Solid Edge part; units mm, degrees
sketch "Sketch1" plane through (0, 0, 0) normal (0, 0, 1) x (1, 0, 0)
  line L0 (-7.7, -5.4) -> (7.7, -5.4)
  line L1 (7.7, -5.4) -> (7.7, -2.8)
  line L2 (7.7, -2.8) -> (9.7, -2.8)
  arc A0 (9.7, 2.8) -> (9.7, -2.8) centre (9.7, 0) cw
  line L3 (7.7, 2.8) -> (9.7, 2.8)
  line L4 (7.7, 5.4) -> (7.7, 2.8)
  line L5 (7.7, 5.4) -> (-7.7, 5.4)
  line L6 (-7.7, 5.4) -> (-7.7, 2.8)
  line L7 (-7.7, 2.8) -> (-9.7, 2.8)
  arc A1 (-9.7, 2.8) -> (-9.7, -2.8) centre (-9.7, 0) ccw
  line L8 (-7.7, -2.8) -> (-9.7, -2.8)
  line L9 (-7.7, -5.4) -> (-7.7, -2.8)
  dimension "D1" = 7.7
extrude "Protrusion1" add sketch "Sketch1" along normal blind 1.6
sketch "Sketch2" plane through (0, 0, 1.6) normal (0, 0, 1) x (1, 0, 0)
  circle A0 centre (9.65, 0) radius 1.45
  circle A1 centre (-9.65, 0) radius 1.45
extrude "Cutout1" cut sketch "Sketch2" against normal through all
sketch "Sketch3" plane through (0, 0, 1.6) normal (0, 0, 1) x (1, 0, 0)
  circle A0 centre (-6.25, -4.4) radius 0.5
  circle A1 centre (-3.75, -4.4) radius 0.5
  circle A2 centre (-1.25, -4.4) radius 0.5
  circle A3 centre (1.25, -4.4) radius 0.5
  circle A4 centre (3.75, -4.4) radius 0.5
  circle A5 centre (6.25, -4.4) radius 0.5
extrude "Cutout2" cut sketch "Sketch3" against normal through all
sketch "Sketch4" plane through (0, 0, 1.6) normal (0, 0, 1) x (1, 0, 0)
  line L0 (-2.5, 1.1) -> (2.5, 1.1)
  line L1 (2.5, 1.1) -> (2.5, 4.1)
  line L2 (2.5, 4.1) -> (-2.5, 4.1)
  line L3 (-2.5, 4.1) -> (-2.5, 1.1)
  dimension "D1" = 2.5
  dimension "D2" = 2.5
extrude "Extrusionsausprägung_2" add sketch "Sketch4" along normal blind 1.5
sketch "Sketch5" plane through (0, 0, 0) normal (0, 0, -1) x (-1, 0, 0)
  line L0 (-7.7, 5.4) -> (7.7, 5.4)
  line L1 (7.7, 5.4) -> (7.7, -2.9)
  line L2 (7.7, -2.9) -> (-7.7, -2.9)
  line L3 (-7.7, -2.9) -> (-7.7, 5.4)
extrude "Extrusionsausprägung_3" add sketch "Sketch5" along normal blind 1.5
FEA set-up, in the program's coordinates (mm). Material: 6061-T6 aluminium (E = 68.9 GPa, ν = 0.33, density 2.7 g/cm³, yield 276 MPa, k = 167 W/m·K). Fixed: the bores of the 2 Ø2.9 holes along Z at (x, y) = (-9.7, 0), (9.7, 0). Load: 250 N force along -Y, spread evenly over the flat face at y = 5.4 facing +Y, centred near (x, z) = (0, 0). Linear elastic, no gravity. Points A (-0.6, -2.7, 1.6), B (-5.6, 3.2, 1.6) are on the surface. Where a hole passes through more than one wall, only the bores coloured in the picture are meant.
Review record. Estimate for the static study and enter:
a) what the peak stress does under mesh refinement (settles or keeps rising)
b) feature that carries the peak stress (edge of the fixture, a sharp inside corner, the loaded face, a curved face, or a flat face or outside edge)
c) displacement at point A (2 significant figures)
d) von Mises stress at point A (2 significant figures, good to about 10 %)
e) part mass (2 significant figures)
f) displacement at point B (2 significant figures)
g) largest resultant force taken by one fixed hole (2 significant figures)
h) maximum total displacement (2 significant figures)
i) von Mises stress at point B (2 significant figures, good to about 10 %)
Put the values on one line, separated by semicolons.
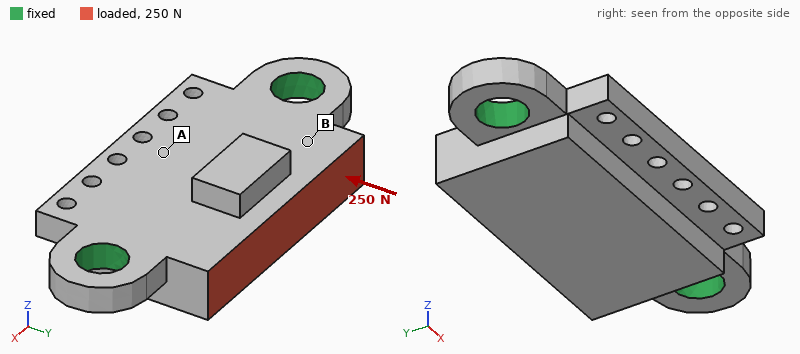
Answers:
keeps rising; edge of the fixture; 2.0 µm; 5.8 MPa; 1.4 g; 2.1 µm; 130 N; 5.0 µm; 10 MPa
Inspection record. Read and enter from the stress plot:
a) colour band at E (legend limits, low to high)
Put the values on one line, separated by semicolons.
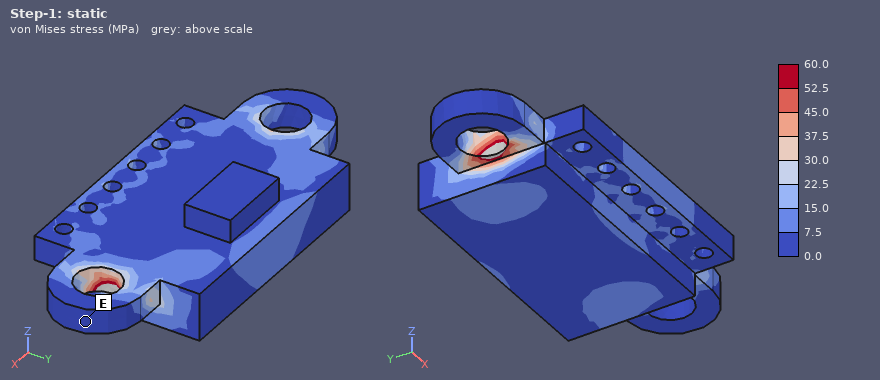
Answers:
0.0 to 7.5 MPa
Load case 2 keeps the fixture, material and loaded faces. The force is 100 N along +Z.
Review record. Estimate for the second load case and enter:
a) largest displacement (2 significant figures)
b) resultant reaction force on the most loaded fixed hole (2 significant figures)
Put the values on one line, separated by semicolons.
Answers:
15 µm; 66 N
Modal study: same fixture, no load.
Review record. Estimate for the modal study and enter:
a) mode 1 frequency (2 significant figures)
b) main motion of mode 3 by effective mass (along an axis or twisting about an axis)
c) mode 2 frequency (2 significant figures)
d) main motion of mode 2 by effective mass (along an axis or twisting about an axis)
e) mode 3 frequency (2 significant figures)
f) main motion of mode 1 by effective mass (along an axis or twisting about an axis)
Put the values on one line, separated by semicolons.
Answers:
24 kHz; along Y; 30 kHz; along Z; 49 kHz; along Z
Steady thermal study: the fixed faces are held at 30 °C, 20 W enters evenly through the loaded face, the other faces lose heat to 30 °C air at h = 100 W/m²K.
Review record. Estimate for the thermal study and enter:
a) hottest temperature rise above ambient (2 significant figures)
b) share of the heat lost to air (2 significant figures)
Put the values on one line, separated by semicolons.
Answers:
27 K; 3.8 %
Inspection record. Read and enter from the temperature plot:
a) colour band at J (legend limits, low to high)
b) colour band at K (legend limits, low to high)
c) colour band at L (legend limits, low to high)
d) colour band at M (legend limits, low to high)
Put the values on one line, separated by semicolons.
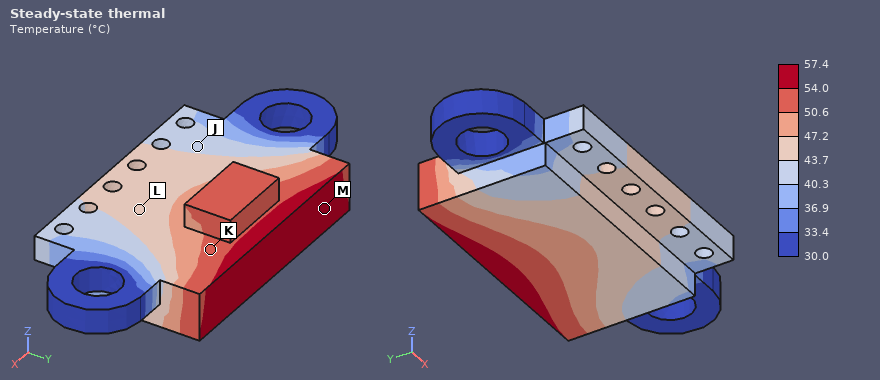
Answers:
40.3 to 43.7 °C; 50.6 to 54.0 °C; 43.7 to 47.2 °C; 54.0 to 57.4 °C
